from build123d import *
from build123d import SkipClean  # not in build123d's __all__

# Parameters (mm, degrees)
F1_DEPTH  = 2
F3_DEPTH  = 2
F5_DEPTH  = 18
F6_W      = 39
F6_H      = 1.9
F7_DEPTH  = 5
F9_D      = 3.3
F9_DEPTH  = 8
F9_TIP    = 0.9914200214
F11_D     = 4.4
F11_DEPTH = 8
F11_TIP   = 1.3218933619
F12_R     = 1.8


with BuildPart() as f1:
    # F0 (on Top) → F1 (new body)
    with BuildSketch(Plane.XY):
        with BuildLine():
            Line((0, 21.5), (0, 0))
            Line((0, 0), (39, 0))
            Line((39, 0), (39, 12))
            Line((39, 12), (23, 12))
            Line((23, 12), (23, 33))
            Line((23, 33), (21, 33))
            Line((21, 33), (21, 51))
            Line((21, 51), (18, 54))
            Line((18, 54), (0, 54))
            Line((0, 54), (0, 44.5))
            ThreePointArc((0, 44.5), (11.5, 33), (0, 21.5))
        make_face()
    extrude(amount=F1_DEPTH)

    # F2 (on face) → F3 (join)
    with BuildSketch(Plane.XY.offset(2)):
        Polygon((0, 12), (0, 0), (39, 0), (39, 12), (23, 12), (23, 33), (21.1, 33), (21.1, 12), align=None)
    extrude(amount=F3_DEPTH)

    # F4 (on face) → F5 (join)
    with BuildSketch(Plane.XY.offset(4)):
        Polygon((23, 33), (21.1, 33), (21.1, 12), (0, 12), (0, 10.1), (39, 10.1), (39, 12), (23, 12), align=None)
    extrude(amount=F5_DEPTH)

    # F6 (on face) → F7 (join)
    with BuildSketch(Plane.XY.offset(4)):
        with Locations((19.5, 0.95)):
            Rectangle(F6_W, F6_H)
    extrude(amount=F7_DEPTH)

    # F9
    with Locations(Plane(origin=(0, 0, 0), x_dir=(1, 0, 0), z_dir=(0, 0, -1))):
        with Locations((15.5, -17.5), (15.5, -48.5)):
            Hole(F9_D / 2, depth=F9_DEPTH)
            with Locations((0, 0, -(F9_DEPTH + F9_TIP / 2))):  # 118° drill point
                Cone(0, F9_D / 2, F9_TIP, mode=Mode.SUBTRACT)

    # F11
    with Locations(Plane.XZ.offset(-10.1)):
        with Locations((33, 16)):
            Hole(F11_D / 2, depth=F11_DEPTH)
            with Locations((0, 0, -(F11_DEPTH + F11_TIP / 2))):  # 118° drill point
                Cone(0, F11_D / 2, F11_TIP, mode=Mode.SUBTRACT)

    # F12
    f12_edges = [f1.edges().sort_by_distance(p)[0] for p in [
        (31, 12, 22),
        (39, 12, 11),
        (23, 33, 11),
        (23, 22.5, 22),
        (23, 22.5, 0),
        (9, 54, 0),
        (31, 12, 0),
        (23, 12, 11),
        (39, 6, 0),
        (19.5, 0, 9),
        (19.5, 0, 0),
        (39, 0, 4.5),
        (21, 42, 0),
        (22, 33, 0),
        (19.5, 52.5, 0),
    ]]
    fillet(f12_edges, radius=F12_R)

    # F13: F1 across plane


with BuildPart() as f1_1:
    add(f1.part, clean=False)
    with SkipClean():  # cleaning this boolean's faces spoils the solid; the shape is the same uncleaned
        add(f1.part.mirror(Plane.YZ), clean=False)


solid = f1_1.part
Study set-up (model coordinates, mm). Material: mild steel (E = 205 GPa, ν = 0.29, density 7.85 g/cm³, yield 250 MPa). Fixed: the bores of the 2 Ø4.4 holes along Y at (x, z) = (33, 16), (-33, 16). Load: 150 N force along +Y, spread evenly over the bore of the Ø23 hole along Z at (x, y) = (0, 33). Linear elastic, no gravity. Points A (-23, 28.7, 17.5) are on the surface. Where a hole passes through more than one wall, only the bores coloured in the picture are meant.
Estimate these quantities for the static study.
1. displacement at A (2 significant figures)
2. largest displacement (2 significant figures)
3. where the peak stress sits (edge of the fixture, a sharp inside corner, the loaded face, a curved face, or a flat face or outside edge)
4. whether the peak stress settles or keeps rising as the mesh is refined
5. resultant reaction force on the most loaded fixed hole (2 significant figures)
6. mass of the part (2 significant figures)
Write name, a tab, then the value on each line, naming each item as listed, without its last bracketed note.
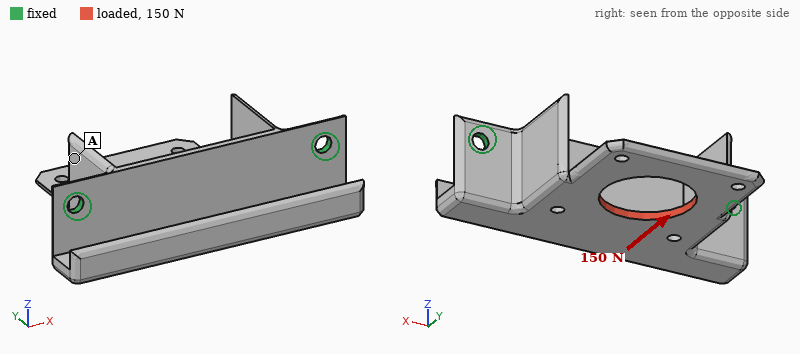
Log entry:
displacement at A	27 µm
largest displacement	71 µm
where the peak stress sits	edge of the fixture
whether the peak stress settles or keeps rising as the mesh is refined	keeps rising
resultant reaction force on the most loaded fixed hole	75 N
mass of the part	88 g
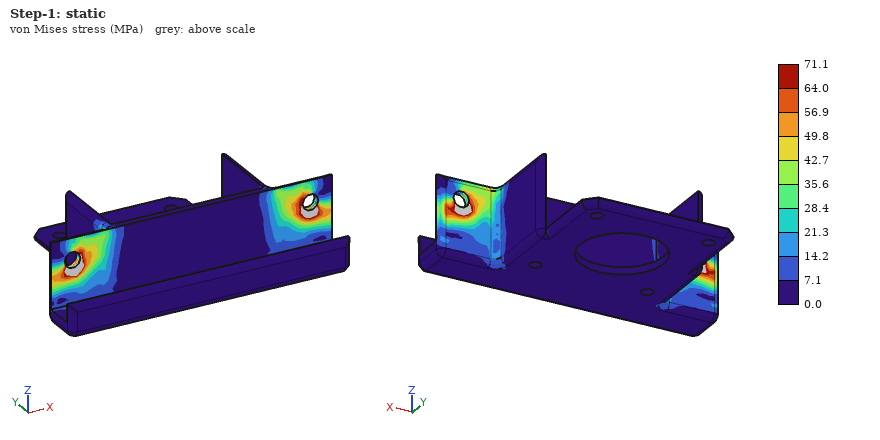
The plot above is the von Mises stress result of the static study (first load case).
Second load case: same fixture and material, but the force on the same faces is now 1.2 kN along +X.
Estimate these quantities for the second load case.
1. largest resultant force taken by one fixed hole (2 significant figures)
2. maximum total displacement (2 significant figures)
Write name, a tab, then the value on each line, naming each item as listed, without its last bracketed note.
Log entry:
largest resultant force taken by one fixed hole	770 N
maximum total displacement	0.12 mm
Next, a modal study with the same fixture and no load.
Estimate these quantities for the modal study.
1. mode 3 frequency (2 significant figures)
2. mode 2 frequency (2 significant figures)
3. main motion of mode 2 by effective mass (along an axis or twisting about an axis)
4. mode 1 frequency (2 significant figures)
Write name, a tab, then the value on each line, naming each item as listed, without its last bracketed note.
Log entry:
mode 3 frequency	2600 Hz
mode 2 frequency	2300 Hz
main motion of mode 2 by effective mass	along Y
mode 1 frequency	990 Hz
